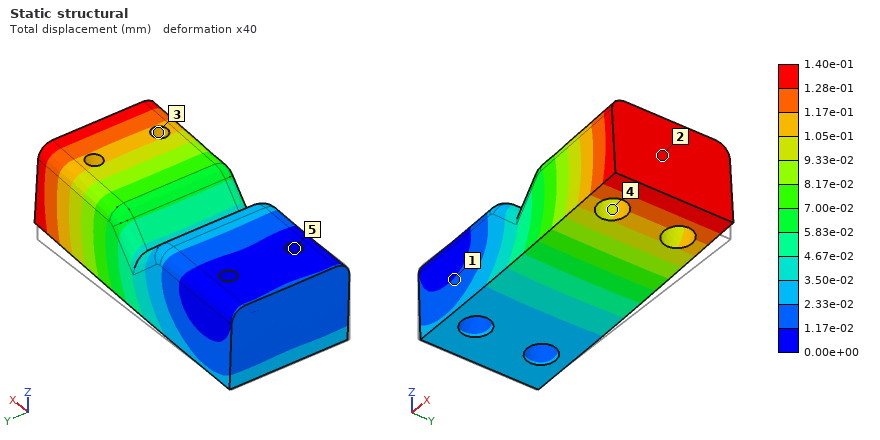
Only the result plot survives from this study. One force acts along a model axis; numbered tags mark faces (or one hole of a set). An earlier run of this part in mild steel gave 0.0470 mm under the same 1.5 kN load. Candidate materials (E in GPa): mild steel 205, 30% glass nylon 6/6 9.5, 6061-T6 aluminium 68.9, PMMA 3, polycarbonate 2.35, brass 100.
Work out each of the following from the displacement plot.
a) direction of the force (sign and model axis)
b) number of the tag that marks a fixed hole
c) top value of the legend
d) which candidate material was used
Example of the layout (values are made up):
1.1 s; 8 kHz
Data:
+Z; 5; 1.40e-01 mm; 6061-T6 aluminium
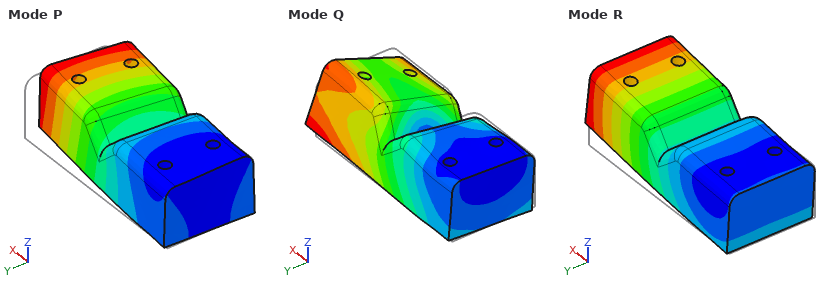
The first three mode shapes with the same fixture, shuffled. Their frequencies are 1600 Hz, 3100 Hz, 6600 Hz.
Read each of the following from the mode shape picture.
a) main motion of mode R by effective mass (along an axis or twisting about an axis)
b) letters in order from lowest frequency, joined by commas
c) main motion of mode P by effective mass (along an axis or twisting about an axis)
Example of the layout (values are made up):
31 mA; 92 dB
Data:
along Z; R, P, Q; along Y
